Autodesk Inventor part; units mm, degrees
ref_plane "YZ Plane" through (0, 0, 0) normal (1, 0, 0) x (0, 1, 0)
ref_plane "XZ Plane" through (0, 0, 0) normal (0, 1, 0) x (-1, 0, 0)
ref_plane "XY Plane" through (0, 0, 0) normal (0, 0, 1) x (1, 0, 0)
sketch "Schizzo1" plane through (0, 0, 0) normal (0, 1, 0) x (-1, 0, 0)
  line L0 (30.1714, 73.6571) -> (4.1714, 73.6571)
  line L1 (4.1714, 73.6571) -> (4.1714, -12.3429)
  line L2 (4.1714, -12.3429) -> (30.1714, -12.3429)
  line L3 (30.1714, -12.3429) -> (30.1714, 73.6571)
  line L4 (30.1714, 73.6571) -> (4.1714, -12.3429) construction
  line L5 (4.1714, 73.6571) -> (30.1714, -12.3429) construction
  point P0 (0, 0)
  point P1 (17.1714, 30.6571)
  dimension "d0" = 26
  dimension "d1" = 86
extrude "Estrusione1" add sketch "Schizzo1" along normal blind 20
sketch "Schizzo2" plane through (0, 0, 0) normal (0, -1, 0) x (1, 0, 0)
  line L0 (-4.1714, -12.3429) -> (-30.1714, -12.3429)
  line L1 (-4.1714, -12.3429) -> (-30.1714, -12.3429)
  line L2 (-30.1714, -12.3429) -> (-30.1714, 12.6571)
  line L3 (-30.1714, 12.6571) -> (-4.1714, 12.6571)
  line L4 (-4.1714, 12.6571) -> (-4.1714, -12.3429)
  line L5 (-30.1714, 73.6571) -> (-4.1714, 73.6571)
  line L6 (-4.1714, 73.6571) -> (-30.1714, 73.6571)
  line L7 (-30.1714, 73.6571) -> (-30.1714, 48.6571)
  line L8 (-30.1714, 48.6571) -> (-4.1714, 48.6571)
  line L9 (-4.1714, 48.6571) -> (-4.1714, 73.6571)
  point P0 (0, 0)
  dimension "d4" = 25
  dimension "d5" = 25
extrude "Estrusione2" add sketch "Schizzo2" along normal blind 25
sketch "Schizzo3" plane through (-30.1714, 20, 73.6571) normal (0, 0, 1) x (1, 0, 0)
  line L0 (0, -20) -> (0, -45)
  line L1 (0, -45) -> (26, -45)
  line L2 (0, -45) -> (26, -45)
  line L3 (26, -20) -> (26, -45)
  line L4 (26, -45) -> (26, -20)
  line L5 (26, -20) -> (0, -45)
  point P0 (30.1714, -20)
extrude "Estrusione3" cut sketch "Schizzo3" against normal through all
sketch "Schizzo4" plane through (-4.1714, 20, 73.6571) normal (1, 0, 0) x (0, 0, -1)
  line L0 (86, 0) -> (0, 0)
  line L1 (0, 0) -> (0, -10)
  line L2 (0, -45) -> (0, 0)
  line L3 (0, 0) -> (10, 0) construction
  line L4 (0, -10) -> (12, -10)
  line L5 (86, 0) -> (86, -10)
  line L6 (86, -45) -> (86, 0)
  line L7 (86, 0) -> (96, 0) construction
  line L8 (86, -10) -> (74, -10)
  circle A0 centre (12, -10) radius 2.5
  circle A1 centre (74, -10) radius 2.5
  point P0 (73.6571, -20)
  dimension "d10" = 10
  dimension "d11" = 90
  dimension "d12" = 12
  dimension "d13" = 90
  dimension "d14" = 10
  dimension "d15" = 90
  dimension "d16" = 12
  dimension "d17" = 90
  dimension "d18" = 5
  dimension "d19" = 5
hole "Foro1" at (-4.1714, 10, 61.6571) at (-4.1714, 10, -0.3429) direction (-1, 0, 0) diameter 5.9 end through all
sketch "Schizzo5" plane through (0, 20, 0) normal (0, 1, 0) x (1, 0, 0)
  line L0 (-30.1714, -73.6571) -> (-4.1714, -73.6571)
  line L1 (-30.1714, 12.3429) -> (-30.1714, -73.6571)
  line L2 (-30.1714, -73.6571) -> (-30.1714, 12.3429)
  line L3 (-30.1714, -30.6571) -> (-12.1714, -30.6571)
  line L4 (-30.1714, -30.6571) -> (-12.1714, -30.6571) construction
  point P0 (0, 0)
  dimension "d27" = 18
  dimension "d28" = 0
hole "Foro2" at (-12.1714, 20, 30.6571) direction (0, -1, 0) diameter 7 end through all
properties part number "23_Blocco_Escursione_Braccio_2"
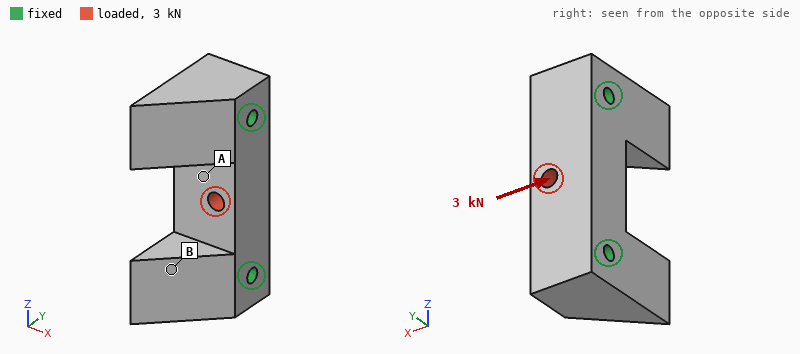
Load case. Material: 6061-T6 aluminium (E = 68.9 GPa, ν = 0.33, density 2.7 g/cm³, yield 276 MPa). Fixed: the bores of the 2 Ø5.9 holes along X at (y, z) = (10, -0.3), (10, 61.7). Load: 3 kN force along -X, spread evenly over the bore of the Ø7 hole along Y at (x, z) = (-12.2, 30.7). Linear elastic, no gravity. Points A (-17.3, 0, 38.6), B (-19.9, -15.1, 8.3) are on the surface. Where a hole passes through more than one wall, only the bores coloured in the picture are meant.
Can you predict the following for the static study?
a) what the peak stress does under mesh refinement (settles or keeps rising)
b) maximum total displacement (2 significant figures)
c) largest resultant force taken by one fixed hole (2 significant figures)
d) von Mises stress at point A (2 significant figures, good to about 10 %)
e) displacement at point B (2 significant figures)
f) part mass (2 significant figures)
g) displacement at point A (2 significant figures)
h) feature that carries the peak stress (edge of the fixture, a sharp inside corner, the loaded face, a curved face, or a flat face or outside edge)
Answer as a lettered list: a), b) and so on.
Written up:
a) keeps rising
b) 6.6 µm
c) 1.5 kN
d) 7.4 MPa
e) 1.1 µm
f) 160 g
g) 4.4 µm
h) edge of the fixture
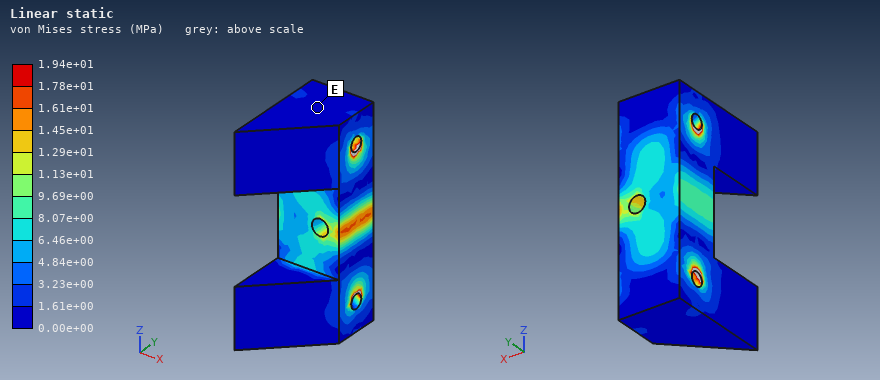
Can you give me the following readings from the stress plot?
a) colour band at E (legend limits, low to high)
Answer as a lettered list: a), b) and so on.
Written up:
a) 0.00e+00 to 1.61e+00 MPa
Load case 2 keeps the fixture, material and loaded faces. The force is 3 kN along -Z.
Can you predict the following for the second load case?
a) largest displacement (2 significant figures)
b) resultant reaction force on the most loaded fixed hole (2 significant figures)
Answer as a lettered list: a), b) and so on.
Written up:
a) 2.0 µm
b) 1.5 kN
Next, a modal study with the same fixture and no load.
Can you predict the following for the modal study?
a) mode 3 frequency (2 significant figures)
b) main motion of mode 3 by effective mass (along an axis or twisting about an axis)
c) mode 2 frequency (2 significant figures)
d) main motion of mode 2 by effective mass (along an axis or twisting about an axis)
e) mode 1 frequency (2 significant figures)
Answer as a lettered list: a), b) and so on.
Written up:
a) 18 kHz
b) along X
c) 17 kHz
d) along Z
e) 11 kHz
